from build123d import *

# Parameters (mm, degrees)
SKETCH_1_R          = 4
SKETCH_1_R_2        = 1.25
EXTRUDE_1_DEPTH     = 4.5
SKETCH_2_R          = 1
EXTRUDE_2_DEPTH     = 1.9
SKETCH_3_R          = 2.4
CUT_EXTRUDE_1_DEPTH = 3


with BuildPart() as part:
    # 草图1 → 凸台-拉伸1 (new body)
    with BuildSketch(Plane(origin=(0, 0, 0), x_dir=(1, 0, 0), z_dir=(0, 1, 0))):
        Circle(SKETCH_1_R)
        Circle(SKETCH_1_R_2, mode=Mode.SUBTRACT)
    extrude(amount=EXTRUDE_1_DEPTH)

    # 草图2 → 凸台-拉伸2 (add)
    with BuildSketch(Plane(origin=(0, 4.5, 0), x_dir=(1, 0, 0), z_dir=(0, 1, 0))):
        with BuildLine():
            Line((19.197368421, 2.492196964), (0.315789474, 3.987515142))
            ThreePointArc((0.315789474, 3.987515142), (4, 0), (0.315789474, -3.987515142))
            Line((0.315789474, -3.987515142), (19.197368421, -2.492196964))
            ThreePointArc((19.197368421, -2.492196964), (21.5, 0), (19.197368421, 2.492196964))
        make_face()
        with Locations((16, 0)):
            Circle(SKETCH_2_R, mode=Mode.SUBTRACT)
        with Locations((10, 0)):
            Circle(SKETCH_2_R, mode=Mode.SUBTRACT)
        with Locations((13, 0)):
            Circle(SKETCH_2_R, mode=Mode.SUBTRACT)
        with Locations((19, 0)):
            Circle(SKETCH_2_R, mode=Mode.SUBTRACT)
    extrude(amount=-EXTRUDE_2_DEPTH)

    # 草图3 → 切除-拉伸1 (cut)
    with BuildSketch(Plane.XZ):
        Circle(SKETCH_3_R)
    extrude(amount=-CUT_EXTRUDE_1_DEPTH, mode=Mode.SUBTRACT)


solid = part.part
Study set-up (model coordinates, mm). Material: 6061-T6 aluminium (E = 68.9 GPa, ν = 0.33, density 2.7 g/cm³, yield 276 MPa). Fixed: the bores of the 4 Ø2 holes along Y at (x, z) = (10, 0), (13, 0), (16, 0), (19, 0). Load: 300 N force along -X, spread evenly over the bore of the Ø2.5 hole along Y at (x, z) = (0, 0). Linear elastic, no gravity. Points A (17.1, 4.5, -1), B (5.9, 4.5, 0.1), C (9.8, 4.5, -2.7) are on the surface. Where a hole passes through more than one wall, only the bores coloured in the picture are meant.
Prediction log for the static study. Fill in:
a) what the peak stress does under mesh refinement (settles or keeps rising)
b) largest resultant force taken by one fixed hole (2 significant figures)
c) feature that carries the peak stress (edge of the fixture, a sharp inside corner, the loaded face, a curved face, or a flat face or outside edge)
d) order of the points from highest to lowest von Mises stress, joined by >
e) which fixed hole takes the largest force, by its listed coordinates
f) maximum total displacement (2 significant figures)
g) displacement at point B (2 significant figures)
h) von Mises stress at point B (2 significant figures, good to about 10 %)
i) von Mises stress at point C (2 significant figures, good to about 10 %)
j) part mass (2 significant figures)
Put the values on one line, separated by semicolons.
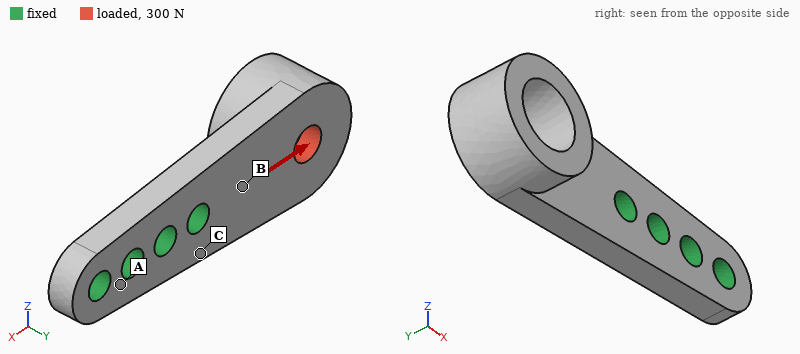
keeps rising; 240 N; edge of the fixture; B > C > A; (10, 0); 18 µm; 2.8 µm; 39 MPa; 21 MPa; 0.94 g
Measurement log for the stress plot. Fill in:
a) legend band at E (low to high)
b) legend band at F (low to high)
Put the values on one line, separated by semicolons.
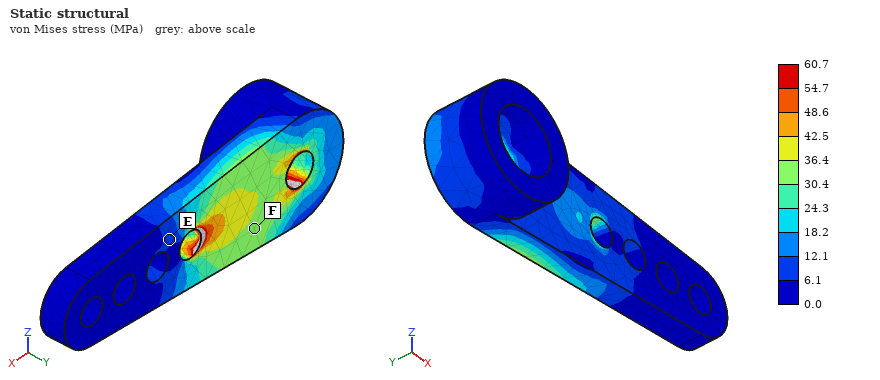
6.1 to 12.1 MPa; 30.4 to 36.4 MPa
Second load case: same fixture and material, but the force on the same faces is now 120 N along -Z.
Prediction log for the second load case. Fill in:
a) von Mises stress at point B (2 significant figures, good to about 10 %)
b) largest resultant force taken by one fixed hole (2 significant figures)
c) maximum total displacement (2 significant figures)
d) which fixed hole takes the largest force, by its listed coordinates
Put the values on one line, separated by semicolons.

32 MPa; 260 N; 34 µm; (10, 0)
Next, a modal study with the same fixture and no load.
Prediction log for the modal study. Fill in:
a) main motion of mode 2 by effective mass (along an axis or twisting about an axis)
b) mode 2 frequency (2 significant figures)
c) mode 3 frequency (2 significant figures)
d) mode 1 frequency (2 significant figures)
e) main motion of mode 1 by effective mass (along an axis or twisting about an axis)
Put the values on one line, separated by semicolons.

along Z; 15 kHz; 21 kHz; 6600 Hz; along Y
